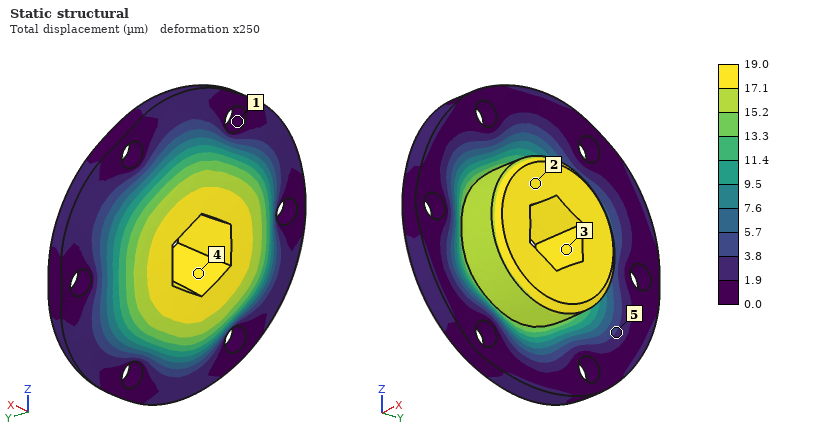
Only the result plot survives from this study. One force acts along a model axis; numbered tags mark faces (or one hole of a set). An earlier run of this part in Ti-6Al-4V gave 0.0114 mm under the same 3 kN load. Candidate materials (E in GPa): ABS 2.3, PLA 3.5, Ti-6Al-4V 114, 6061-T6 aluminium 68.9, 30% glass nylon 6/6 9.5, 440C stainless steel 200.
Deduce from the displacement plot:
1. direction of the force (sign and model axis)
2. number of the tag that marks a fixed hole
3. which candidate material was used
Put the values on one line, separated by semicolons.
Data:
-X; 1; 6061-T6 aluminium
